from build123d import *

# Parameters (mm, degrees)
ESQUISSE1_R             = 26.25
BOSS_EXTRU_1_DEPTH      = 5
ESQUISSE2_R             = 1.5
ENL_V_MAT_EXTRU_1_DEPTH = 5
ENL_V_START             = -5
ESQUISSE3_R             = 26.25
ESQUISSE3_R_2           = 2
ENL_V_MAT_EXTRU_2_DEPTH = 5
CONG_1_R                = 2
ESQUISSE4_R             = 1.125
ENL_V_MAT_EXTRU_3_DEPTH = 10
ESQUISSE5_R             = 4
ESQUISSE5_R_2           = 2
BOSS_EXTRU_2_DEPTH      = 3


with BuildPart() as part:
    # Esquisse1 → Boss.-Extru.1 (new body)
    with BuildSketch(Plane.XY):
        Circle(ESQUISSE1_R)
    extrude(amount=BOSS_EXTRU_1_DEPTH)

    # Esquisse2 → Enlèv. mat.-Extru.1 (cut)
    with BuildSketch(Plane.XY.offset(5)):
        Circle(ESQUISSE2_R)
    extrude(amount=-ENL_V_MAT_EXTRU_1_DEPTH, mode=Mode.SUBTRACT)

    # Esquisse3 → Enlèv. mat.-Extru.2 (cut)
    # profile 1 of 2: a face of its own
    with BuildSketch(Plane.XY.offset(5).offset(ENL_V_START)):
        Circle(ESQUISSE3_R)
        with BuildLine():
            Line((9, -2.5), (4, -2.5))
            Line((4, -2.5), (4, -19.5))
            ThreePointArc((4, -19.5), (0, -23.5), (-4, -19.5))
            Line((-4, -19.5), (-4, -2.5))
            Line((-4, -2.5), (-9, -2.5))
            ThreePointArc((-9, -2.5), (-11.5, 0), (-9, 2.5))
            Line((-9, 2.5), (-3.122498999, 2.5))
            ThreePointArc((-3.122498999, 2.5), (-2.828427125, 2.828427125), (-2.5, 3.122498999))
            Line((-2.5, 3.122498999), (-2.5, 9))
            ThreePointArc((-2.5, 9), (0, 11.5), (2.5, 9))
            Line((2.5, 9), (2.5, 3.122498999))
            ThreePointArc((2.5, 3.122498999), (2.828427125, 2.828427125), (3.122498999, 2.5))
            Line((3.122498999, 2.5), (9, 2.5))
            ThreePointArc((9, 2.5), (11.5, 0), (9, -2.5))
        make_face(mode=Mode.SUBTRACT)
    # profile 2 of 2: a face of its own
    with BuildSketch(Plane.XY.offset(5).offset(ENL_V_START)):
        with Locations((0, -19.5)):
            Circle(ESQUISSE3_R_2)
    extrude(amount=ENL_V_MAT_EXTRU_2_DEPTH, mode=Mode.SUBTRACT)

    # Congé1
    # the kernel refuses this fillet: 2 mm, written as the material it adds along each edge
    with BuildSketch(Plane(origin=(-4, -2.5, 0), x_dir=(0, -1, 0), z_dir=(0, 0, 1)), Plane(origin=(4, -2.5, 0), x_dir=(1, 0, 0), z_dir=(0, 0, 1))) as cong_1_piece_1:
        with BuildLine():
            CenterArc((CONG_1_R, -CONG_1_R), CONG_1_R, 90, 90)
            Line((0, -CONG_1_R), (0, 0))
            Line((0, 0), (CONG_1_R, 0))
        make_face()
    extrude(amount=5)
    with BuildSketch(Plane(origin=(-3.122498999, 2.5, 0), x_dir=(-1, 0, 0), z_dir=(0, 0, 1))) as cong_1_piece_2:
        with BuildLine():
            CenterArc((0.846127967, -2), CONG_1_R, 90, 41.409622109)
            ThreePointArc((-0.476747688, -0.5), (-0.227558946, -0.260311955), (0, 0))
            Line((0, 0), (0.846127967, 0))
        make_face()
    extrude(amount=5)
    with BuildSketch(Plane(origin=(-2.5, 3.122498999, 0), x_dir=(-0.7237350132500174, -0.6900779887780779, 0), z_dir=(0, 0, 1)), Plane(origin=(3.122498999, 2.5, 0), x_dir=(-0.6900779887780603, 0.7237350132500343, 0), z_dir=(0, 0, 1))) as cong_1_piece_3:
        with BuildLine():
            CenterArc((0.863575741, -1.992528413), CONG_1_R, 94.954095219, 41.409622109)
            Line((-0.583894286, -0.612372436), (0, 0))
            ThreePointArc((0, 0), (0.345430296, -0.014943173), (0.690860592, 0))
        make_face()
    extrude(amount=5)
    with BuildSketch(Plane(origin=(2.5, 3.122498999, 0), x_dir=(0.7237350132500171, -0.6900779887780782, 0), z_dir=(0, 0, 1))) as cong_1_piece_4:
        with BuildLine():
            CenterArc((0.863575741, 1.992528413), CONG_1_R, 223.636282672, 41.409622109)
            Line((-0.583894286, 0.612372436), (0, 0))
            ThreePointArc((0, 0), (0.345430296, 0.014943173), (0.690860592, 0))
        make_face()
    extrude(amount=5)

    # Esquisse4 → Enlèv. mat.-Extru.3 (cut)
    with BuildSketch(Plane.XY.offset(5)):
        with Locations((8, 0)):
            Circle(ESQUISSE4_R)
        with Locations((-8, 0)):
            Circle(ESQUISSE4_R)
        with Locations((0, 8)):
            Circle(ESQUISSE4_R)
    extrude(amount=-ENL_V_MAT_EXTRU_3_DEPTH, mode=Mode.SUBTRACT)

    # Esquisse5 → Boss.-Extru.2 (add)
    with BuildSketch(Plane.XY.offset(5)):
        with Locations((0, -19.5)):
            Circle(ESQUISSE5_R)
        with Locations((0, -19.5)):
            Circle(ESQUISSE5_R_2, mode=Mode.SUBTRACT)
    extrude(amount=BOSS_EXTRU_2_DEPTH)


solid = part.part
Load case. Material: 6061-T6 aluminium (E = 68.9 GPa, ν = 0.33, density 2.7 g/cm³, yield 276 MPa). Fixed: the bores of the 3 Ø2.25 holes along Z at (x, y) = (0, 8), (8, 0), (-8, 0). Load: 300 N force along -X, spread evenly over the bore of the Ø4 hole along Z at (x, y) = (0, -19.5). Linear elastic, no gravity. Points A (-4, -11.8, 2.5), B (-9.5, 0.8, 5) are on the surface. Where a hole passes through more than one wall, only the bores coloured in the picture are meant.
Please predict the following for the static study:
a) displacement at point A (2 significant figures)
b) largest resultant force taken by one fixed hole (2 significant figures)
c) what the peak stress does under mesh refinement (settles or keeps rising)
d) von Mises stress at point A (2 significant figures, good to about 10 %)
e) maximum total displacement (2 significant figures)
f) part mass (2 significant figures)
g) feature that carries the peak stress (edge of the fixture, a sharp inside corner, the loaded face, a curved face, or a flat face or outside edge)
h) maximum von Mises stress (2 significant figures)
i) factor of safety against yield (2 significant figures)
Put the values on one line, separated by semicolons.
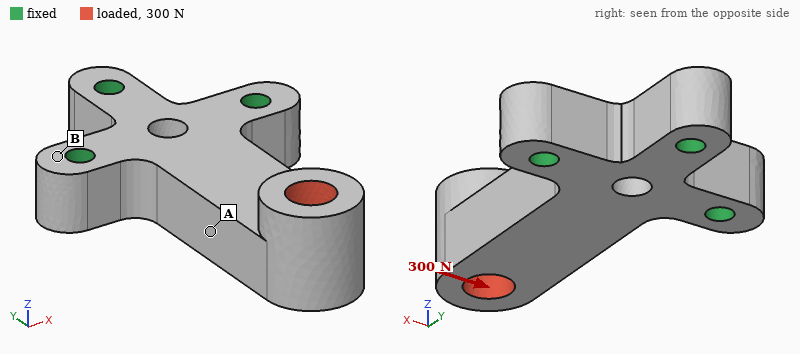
26 µm; 430 N; settles; 46 MPa; 76 µm; 4.1 g; a curved face; 140 MPa; 1.9
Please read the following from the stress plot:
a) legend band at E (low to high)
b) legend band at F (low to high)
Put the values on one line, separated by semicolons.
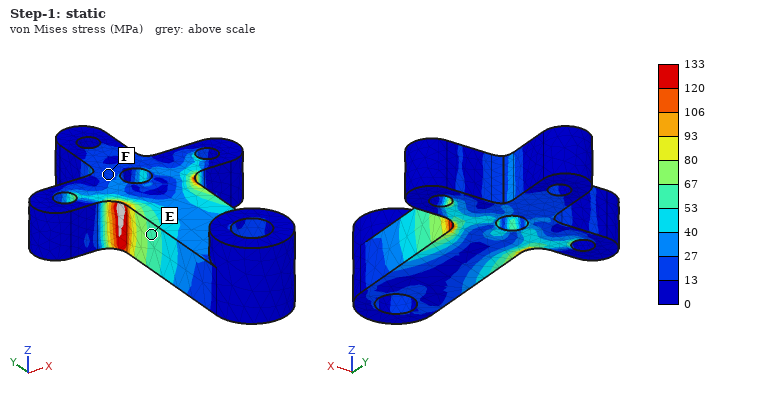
53 to 67 MPa; 13 to 27 MPa
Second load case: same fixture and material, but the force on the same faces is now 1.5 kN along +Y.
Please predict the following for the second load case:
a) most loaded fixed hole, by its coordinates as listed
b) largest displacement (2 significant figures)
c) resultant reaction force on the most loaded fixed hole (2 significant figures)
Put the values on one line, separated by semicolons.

(0, 8); 0.14 mm; 690 N
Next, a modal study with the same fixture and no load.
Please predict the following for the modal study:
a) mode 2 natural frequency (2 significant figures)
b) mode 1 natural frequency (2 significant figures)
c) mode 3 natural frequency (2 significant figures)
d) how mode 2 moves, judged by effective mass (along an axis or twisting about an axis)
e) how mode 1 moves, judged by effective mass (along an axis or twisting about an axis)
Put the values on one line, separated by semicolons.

11 kHz; 5900 Hz; 25 kHz; along X; along Z
